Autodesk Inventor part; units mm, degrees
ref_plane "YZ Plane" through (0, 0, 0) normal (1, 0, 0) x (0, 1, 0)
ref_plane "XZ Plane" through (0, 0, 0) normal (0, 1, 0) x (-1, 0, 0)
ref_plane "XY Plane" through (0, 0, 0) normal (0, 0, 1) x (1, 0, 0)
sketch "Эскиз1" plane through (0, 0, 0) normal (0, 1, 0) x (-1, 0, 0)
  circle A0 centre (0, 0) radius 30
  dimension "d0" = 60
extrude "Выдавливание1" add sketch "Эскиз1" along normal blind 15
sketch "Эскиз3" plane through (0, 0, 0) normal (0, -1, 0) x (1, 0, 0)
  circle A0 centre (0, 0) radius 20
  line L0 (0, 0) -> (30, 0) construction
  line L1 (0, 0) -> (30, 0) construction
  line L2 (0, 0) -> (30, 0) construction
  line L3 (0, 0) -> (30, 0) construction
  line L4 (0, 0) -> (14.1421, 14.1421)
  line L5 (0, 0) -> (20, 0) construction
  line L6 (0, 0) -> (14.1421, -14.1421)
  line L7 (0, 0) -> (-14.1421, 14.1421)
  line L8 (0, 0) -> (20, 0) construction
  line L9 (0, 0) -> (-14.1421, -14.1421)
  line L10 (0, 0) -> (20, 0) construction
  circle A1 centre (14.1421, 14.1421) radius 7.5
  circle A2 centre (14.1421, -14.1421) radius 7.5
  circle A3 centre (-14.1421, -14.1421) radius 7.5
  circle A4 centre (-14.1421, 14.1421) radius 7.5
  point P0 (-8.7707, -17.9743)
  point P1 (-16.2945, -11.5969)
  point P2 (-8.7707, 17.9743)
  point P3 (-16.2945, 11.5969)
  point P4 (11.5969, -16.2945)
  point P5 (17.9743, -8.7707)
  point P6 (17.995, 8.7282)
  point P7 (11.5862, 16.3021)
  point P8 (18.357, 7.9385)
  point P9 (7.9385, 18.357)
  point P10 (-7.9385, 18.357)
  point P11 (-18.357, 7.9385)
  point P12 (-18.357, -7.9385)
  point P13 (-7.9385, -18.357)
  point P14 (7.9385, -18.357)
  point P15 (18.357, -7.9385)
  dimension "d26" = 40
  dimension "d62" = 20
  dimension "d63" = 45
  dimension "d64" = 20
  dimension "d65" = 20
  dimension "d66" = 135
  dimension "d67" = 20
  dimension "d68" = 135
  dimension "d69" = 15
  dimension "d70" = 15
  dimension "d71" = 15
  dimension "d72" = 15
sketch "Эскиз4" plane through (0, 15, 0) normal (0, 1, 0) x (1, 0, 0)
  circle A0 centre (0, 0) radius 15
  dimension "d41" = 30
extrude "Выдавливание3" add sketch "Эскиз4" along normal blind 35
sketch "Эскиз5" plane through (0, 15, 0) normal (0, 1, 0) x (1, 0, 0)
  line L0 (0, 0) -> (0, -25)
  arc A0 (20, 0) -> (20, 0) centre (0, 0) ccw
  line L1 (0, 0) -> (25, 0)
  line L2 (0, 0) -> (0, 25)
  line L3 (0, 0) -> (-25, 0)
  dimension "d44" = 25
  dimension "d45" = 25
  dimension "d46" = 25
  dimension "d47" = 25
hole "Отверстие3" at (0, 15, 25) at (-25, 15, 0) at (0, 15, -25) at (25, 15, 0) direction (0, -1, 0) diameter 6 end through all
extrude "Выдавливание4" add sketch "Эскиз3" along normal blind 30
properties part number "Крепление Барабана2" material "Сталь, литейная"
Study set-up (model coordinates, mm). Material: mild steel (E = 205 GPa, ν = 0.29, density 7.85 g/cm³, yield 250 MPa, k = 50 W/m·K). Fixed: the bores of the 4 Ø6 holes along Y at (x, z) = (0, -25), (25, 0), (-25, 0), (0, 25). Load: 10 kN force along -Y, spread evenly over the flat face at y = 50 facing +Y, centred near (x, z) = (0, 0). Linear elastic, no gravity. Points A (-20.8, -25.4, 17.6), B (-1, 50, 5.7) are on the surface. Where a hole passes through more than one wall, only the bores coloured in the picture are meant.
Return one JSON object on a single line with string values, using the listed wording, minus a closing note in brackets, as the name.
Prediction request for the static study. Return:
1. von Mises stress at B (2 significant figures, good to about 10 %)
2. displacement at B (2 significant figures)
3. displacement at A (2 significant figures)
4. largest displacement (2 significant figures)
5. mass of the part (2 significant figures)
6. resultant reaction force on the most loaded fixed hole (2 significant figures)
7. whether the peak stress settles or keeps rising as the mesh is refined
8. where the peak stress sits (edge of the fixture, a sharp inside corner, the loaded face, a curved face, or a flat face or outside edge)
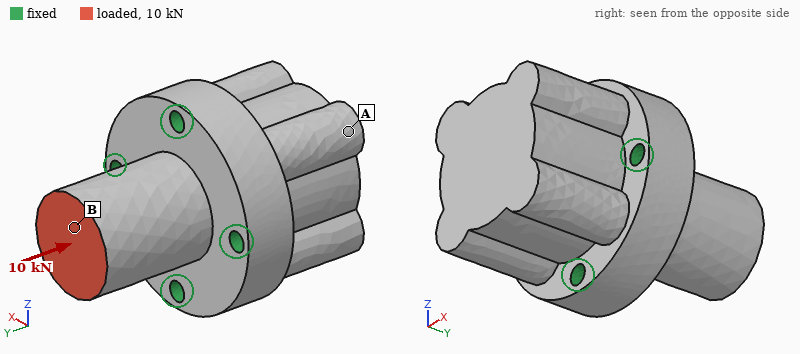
{"von Mises stress at B": "14 MPa", "displacement at B": "3.9 µm", "displacement at A": "0.94 µm", "largest displacement": "4.0 µm", "mass of the part": "900 g", "resultant reaction force on the most loaded fixed hole": "2.5 kN", "whether the peak stress settles or keeps rising as the mesh is refined": "keeps rising", "where the peak stress sits": "edge of the fixture"}
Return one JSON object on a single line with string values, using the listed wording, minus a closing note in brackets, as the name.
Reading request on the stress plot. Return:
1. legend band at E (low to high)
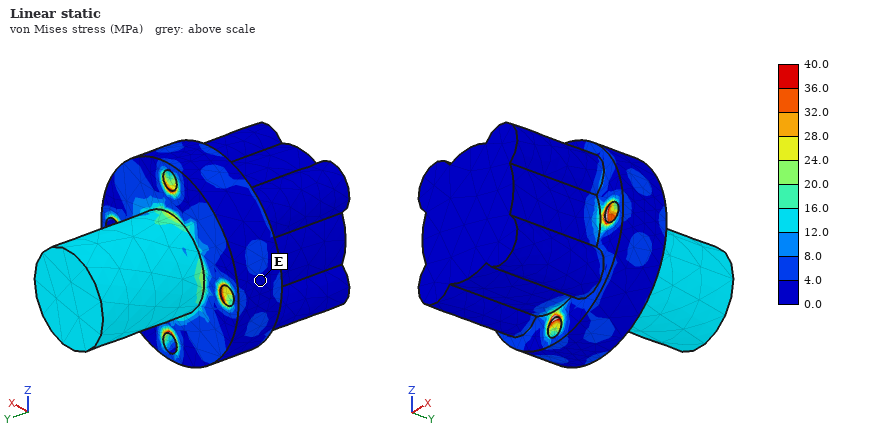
{"legend band at E": "0.0 to 4.0 MPa"}
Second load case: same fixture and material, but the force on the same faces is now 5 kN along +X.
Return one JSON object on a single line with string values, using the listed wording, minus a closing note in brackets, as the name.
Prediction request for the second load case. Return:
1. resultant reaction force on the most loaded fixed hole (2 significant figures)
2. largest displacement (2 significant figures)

{"resultant reaction force on the most loaded fixed hole": "4.5 kN", "largest displacement": "22 µm"}
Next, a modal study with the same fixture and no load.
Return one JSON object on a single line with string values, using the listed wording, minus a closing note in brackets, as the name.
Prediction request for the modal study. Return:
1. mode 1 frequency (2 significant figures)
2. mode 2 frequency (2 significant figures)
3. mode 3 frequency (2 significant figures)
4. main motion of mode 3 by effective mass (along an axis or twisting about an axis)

{"mode 1 frequency": "9300 Hz", "mode 2 frequency": "9300 Hz", "mode 3 frequency": "13 kHz", "main motion of mode 3 by effective mass": "along X"}
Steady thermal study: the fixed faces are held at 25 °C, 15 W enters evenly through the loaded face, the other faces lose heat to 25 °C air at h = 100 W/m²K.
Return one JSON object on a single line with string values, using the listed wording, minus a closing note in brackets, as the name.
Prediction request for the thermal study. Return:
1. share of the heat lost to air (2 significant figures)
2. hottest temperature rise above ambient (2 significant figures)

{"share of the heat lost to air": "28 %", "hottest temperature rise above ambient": "16 K"}
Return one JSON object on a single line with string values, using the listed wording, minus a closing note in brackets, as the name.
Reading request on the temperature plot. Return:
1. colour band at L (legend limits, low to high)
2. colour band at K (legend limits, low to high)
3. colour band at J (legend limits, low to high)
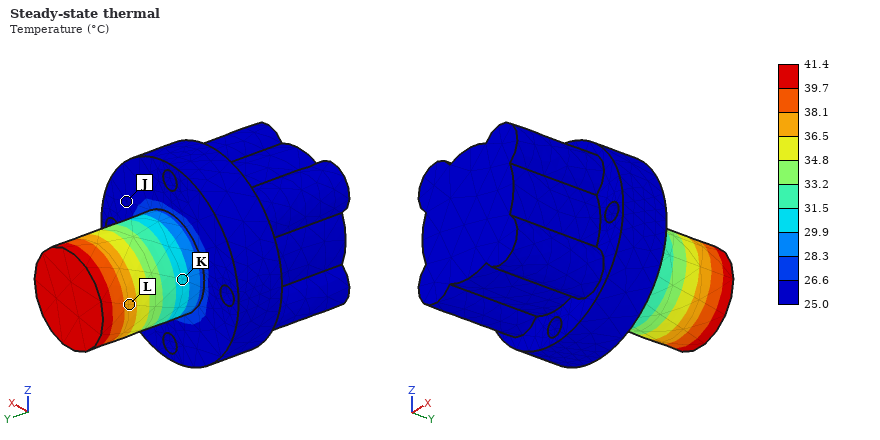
{"colour band at L": "36.5 to 38.1 °C", "colour band at K": "29.9 to 31.5 °C", "colour band at J": "25.0 to 26.6 °C"}
